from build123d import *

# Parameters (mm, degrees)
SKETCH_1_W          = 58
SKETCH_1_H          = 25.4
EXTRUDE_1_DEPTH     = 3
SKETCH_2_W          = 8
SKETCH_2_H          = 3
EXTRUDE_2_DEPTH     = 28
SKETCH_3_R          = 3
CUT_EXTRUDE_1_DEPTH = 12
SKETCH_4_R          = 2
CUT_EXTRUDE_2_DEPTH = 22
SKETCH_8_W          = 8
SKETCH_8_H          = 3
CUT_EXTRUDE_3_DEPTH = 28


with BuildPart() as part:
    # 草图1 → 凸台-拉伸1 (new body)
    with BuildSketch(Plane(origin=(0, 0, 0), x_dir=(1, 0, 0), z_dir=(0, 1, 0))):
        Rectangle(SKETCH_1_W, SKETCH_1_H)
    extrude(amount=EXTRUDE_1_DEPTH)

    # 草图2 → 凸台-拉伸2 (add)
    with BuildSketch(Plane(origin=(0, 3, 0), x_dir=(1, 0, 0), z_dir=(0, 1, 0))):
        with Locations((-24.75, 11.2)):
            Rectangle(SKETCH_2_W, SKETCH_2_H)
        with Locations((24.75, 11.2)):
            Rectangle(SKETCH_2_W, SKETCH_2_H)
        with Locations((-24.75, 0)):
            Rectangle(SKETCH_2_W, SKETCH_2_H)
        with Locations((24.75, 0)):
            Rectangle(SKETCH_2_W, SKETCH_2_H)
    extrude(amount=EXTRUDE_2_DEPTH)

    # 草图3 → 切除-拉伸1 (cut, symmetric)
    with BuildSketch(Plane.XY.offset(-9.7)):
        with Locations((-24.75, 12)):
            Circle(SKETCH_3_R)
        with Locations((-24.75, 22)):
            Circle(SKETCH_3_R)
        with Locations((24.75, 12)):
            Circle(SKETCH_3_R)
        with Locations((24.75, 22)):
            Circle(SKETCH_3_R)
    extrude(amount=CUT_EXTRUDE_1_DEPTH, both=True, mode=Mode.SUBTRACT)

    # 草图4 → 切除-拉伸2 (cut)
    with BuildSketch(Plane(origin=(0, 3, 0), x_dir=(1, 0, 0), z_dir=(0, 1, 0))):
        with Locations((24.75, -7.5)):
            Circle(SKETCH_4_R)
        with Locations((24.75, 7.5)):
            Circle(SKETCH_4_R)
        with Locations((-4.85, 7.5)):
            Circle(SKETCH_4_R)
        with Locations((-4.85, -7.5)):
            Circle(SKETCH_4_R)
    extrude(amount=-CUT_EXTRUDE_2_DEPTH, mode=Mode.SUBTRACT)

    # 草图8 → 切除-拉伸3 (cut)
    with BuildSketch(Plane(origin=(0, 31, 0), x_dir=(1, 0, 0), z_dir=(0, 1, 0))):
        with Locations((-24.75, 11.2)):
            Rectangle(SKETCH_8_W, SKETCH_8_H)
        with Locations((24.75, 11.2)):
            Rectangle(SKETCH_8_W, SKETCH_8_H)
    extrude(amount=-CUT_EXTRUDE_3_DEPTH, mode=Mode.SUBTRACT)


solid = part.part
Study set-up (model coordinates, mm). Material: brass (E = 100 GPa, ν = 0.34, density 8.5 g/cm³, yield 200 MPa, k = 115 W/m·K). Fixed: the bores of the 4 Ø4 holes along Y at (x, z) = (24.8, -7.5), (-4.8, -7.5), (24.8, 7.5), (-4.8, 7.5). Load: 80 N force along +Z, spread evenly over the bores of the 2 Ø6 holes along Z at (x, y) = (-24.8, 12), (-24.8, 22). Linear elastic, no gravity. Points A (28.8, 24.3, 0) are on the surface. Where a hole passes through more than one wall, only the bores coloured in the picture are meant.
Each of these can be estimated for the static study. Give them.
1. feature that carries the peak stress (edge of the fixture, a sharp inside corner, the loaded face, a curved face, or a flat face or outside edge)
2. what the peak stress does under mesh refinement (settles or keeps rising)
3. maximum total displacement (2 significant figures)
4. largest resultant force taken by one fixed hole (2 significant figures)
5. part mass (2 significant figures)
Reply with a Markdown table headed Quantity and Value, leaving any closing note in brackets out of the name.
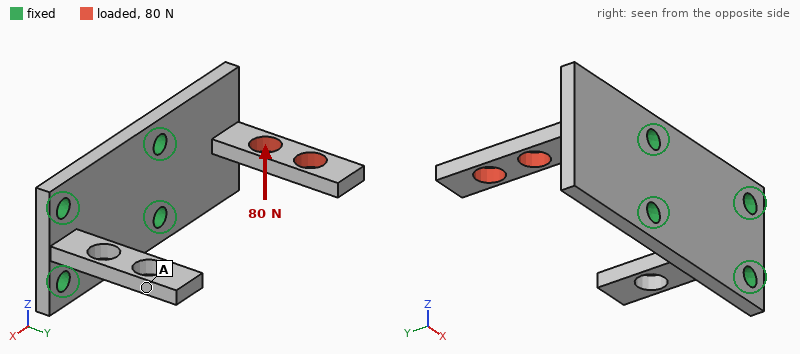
| Quantity | Value |
|---|---|
| feature that carries the peak stress | a sharp inside corner |
| what the peak stress does under mesh refinement | keeps rising |
| maximum total displacement | 0.27 mm |
| largest resultant force taken by one fixed hole | 120 N |
| part mass | 45 g |
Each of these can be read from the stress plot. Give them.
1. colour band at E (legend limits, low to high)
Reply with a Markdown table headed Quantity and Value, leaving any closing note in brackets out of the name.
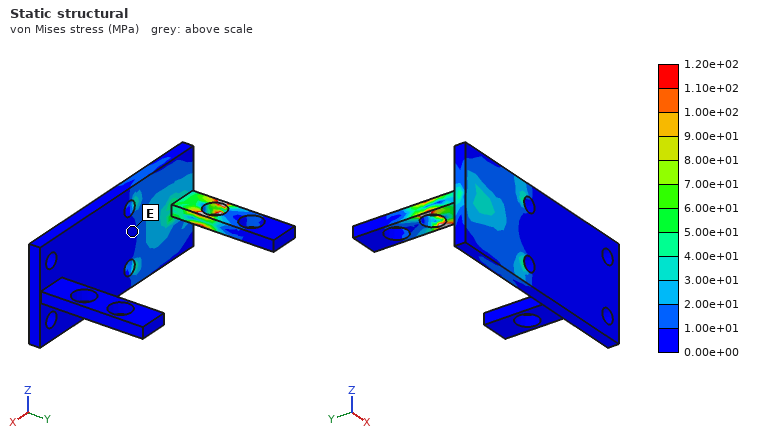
| Quantity | Value |
|---|---|
| colour band at E | 0.00e+00 to 1.00e+01 MPa |
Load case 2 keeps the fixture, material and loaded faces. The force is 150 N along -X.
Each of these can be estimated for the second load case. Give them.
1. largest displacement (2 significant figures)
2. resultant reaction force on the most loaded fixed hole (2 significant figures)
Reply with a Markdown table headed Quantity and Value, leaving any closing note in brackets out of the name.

| Quantity | Value |
|---|---|
| largest displacement | 0.30 mm |
| resultant reaction force on the most loaded fixed hole | 74 N |
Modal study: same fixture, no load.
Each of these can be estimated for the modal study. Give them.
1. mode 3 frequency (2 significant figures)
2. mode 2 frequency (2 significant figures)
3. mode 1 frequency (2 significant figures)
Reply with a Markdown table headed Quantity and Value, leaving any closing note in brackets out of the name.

| Quantity | Value |
|---|---|
| mode 3 frequency | 1700 Hz |
| mode 2 frequency | 1700 Hz |
| mode 1 frequency | 1500 Hz |
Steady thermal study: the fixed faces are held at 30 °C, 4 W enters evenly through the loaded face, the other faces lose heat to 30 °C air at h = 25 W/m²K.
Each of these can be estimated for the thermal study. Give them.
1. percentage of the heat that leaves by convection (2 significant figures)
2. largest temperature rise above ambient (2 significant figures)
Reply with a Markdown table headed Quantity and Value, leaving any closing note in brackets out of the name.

| Quantity | Value |
|---|---|
| percentage of the heat that leaves by convection | 15 % |
| largest temperature rise above ambient | 44 K |
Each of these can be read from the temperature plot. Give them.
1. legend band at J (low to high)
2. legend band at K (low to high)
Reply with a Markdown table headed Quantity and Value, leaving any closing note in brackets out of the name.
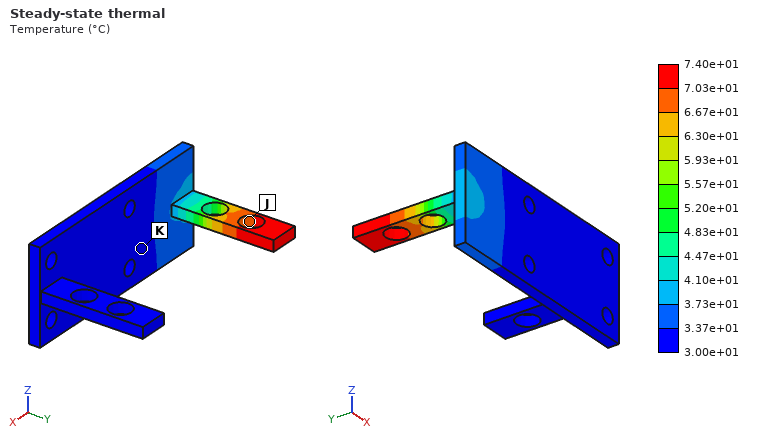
| Quantity | Value |
|---|---|
| legend band at J | 6.67e+01 to 7.03e+01 °C |
| legend band at K | 3.00e+01 to 3.37e+01 °C |
